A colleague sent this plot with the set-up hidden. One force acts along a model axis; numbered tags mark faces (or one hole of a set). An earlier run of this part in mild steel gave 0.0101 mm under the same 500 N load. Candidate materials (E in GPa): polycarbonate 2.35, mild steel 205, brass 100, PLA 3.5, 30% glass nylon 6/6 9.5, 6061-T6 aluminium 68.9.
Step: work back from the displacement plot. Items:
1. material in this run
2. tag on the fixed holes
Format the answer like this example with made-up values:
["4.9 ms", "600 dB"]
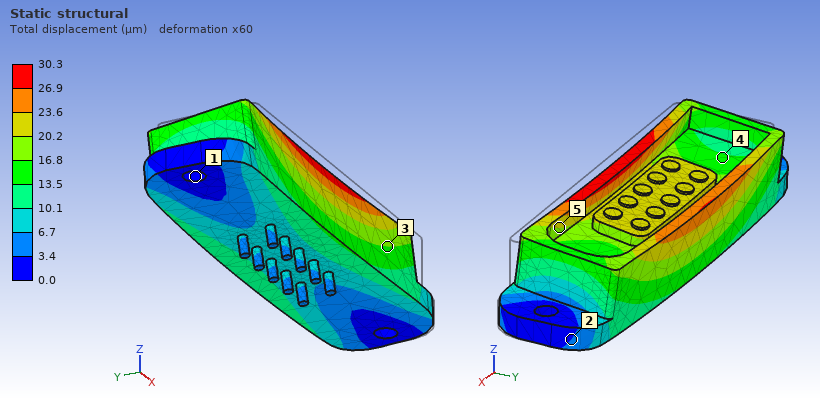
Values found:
["6061-T6 aluminium", "1"]
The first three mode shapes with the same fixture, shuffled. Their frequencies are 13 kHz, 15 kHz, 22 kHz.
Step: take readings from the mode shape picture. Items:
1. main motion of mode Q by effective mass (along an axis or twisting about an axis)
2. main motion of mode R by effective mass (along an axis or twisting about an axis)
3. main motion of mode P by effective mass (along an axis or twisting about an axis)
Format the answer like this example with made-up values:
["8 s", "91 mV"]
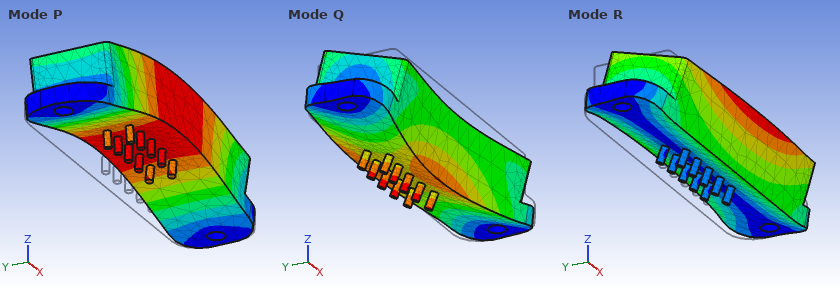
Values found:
["along Y", "along Y", "along Z"]
